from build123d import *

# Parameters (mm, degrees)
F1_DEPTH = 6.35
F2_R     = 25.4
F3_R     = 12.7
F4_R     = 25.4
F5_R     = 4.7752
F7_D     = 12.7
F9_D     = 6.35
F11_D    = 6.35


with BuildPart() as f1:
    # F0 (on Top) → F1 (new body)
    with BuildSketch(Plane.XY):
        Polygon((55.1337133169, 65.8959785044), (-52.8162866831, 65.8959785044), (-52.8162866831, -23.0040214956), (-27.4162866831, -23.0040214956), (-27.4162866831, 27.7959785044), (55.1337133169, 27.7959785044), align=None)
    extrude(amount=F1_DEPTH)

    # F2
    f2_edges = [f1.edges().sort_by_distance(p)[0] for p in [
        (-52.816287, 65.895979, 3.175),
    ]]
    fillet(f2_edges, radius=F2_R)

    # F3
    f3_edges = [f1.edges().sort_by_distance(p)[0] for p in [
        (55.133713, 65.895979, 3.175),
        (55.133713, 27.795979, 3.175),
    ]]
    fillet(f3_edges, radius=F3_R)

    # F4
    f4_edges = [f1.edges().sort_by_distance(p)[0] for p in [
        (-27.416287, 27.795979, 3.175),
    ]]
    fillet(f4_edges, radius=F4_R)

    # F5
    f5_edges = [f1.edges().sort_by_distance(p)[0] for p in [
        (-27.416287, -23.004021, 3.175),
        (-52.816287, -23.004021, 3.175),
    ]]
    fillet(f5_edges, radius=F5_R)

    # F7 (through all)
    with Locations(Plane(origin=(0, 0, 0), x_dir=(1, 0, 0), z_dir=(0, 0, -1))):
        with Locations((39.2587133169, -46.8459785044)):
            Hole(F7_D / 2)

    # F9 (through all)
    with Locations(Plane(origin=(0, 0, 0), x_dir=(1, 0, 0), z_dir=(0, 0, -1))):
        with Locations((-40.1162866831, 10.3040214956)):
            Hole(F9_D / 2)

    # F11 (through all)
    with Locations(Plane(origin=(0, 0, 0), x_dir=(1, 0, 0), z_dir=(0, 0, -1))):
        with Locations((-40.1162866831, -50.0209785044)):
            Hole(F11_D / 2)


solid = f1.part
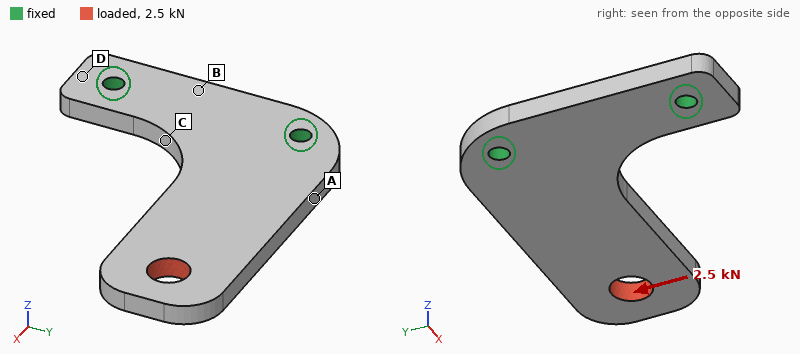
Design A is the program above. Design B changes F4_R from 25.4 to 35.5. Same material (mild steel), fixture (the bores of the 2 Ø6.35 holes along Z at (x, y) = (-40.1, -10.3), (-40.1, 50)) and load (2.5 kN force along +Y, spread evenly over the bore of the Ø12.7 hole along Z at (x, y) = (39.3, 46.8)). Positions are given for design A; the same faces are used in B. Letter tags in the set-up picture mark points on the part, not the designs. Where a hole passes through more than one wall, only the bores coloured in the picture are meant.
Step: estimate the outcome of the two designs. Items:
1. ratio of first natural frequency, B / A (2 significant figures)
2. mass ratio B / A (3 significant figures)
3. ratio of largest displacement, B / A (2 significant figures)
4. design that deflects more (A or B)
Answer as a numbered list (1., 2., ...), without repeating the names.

1. 1.0
2. 1.03
3. 0.79
4. A
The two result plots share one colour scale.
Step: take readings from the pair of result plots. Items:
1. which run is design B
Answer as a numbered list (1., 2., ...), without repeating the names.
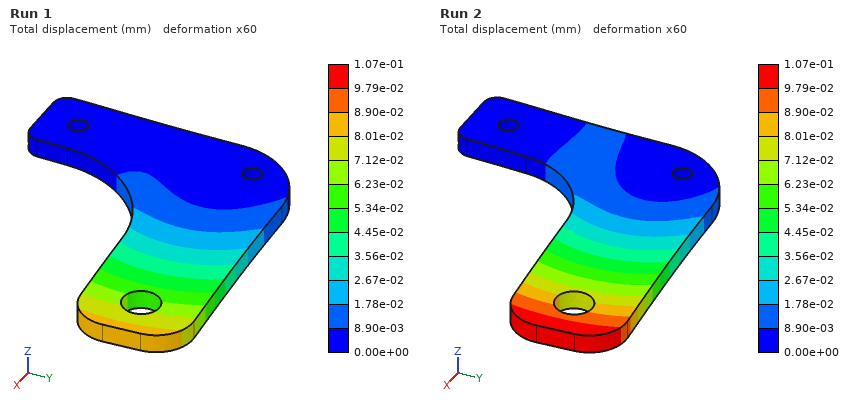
1. Run 1
